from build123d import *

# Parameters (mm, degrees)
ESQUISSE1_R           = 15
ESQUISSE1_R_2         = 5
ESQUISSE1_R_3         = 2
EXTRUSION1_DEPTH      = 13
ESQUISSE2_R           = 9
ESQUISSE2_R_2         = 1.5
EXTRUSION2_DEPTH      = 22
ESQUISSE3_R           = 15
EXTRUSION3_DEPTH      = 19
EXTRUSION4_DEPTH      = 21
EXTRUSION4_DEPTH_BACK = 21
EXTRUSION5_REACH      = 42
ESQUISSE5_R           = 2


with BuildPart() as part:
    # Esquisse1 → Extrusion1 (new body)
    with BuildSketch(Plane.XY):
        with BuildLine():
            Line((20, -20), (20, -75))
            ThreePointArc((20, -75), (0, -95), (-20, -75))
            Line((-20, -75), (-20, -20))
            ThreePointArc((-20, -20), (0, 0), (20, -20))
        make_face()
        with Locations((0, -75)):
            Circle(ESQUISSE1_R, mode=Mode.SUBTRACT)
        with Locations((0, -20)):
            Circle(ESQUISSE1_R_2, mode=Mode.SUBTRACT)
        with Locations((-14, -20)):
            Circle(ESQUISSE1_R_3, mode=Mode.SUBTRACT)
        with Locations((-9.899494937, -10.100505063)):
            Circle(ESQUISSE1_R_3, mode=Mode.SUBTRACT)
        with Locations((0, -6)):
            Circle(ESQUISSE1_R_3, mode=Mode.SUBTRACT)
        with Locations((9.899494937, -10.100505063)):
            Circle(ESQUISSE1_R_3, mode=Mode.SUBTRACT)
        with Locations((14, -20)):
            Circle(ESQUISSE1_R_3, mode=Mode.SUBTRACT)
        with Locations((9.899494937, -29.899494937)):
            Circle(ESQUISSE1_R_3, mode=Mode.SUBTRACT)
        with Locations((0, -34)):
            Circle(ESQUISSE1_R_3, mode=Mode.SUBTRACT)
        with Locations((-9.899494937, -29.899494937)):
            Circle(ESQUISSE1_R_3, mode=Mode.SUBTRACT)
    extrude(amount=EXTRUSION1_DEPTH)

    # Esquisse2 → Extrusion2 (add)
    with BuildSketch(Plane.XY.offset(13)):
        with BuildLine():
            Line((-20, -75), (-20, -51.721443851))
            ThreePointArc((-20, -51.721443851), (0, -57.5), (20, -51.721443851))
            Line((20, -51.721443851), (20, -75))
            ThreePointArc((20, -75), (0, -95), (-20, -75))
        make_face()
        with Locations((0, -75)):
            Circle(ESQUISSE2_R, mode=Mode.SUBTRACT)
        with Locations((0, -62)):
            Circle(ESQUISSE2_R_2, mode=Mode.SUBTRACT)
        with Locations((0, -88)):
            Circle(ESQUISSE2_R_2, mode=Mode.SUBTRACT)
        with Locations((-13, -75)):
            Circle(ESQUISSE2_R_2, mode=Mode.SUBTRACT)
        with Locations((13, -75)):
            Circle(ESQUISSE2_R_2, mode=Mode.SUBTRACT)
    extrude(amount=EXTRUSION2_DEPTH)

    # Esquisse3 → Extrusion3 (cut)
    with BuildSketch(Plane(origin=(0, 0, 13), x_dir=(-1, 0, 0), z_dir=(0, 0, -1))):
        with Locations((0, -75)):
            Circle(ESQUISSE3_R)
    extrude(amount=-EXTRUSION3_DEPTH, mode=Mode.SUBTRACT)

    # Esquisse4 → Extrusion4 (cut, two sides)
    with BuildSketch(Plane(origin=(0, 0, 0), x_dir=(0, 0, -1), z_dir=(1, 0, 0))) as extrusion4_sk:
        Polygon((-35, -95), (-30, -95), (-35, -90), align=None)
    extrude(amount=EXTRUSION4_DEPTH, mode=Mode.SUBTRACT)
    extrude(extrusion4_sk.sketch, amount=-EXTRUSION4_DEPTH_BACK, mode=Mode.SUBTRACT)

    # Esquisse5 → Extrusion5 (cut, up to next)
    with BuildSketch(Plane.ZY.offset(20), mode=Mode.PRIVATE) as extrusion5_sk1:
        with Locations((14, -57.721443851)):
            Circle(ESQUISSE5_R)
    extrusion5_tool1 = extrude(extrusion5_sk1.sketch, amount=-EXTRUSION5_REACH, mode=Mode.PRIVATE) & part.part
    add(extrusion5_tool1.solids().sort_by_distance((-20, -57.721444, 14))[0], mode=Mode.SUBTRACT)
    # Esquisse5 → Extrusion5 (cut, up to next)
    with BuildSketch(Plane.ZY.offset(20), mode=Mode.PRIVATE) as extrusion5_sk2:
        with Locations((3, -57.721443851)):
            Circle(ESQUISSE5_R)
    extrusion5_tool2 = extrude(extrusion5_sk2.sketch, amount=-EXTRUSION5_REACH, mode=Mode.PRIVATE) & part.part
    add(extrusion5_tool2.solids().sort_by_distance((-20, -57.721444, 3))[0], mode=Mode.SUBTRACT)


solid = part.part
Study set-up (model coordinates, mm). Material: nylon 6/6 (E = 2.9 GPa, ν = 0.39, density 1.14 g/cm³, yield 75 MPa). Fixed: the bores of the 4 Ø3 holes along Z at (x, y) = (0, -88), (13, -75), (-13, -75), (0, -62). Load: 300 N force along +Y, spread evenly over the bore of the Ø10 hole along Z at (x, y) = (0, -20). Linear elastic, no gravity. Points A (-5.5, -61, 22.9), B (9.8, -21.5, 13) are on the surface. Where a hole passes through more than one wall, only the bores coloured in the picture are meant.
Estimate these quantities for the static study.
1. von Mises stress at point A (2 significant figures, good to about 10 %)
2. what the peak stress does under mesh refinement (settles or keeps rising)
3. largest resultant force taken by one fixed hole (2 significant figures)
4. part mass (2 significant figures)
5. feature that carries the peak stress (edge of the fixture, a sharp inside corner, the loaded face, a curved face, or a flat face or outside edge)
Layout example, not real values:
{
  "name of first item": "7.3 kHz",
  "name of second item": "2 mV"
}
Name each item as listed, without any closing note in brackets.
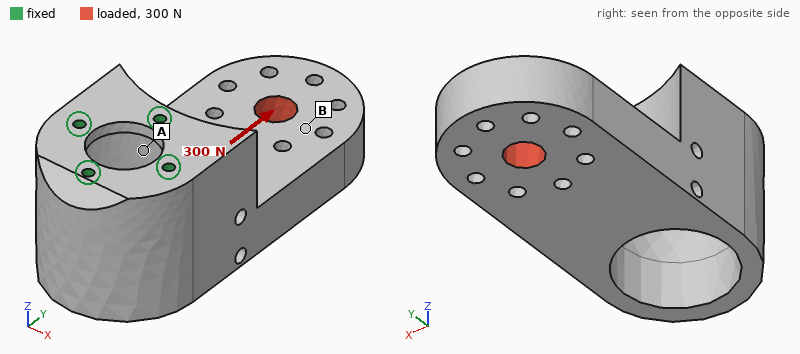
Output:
{
  "von Mises stress at point A": "3.3 MPa",
  "what the peak stress does under mesh refinement": "keeps rising",
  "largest resultant force taken by one fixed hole": "270 N",
  "part mass": "56 g",
  "feature that carries the peak stress": "edge of the fixture"
}
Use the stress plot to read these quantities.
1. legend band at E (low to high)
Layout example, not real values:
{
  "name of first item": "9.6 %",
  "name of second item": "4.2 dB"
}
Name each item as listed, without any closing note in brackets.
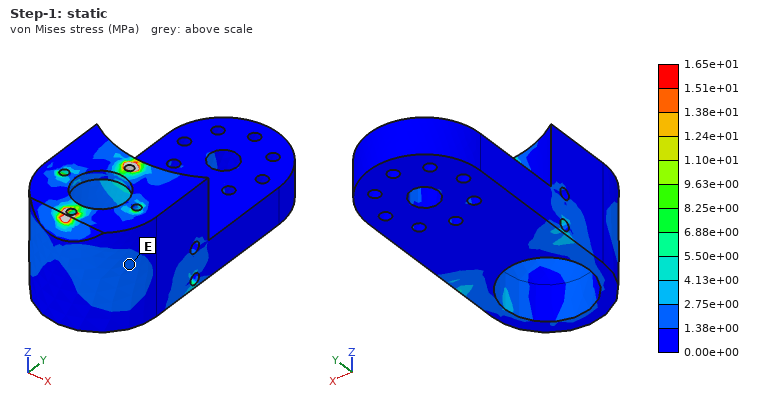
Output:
{
  "legend band at E": "1.38e+00 to 2.75e+00 MPa"
}
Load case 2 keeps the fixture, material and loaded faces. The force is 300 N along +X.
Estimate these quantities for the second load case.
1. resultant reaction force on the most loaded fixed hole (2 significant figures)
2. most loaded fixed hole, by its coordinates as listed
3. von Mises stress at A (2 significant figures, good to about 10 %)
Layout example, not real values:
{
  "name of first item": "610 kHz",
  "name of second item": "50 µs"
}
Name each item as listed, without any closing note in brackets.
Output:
{
  "resultant reaction force on the most loaded fixed hole": "470 N",
  "most loaded fixed hole, by its coordinates as listed": "(0, -62)",
  "von Mises stress at A": "4.9 MPa"
}
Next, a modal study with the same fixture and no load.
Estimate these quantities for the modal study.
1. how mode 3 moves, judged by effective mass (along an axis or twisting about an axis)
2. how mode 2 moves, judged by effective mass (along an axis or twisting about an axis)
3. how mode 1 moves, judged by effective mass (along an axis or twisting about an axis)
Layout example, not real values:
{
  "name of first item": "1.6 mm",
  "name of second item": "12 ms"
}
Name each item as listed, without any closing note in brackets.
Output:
{
  "how mode 3 moves, judged by effective mass": "along Y",
  "how mode 2 moves, judged by effective mass": "along X",
  "how mode 1 moves, judged by effective mass": "along Z"
}
